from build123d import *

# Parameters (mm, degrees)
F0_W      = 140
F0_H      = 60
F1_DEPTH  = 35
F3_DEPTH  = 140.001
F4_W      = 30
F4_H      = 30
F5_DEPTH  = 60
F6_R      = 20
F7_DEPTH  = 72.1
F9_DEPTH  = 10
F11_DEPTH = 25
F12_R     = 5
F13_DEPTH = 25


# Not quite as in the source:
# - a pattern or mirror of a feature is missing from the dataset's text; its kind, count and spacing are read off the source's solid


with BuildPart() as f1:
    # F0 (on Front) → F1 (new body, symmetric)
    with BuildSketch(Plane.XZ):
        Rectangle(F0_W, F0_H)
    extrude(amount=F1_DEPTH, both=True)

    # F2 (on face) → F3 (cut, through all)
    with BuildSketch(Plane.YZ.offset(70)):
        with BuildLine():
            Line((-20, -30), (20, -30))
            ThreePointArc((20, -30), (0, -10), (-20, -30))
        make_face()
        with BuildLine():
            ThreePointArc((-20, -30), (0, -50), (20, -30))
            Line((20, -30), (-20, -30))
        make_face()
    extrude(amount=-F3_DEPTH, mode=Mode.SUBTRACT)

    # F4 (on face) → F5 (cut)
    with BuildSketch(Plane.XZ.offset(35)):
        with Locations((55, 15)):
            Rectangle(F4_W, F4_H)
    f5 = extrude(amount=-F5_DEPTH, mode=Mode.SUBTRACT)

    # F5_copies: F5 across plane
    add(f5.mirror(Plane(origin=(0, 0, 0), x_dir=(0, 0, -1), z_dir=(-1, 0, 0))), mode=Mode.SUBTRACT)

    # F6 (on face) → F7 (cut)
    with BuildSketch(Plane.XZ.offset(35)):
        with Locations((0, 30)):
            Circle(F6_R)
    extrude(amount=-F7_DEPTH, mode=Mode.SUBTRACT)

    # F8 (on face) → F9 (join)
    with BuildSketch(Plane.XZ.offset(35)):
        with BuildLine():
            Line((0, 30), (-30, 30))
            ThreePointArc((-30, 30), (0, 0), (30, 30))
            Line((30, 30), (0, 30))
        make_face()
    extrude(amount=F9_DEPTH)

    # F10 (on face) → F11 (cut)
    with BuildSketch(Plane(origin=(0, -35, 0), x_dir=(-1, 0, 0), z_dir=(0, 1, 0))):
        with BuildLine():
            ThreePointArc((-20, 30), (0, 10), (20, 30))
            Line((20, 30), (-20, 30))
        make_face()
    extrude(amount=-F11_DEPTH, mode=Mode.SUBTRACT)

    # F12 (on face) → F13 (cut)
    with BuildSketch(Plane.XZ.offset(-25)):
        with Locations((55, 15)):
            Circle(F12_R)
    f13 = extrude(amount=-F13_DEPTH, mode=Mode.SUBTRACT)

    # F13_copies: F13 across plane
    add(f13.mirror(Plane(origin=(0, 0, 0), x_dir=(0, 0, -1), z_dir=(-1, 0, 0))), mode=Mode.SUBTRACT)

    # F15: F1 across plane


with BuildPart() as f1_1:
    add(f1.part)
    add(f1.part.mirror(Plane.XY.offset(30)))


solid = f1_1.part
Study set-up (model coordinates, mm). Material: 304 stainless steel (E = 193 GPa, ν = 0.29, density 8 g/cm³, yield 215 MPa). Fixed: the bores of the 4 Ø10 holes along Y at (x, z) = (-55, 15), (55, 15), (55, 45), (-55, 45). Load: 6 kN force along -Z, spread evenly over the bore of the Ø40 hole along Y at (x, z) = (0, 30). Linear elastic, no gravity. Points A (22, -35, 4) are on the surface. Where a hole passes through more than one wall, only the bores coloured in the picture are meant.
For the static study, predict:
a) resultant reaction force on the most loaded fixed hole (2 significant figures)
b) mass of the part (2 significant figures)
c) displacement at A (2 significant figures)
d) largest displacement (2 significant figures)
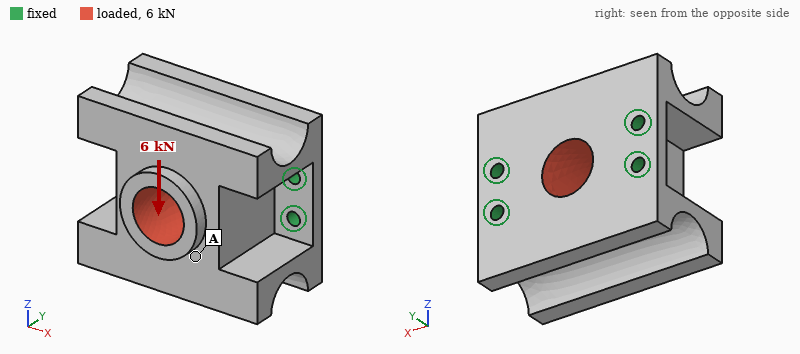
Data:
2.8 kN
5.7 kg
12 µm
15 µm
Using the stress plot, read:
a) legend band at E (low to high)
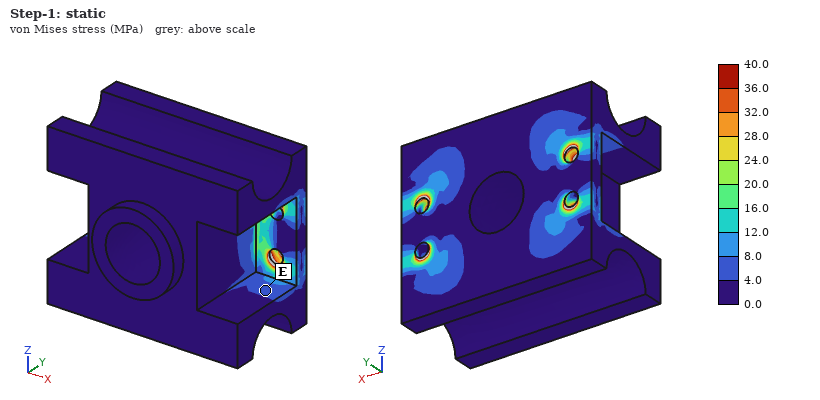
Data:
4.0 to 8.0 MPa
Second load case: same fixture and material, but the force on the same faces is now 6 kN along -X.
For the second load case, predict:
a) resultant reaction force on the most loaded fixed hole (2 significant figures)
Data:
1.8 kN
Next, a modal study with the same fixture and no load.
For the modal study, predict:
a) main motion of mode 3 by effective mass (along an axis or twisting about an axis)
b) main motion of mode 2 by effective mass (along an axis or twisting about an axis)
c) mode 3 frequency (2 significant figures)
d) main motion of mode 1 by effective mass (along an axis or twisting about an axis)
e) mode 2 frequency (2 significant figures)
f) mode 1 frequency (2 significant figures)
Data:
along Y
along X
3700 Hz
along Z
3600 Hz
1500 Hz
